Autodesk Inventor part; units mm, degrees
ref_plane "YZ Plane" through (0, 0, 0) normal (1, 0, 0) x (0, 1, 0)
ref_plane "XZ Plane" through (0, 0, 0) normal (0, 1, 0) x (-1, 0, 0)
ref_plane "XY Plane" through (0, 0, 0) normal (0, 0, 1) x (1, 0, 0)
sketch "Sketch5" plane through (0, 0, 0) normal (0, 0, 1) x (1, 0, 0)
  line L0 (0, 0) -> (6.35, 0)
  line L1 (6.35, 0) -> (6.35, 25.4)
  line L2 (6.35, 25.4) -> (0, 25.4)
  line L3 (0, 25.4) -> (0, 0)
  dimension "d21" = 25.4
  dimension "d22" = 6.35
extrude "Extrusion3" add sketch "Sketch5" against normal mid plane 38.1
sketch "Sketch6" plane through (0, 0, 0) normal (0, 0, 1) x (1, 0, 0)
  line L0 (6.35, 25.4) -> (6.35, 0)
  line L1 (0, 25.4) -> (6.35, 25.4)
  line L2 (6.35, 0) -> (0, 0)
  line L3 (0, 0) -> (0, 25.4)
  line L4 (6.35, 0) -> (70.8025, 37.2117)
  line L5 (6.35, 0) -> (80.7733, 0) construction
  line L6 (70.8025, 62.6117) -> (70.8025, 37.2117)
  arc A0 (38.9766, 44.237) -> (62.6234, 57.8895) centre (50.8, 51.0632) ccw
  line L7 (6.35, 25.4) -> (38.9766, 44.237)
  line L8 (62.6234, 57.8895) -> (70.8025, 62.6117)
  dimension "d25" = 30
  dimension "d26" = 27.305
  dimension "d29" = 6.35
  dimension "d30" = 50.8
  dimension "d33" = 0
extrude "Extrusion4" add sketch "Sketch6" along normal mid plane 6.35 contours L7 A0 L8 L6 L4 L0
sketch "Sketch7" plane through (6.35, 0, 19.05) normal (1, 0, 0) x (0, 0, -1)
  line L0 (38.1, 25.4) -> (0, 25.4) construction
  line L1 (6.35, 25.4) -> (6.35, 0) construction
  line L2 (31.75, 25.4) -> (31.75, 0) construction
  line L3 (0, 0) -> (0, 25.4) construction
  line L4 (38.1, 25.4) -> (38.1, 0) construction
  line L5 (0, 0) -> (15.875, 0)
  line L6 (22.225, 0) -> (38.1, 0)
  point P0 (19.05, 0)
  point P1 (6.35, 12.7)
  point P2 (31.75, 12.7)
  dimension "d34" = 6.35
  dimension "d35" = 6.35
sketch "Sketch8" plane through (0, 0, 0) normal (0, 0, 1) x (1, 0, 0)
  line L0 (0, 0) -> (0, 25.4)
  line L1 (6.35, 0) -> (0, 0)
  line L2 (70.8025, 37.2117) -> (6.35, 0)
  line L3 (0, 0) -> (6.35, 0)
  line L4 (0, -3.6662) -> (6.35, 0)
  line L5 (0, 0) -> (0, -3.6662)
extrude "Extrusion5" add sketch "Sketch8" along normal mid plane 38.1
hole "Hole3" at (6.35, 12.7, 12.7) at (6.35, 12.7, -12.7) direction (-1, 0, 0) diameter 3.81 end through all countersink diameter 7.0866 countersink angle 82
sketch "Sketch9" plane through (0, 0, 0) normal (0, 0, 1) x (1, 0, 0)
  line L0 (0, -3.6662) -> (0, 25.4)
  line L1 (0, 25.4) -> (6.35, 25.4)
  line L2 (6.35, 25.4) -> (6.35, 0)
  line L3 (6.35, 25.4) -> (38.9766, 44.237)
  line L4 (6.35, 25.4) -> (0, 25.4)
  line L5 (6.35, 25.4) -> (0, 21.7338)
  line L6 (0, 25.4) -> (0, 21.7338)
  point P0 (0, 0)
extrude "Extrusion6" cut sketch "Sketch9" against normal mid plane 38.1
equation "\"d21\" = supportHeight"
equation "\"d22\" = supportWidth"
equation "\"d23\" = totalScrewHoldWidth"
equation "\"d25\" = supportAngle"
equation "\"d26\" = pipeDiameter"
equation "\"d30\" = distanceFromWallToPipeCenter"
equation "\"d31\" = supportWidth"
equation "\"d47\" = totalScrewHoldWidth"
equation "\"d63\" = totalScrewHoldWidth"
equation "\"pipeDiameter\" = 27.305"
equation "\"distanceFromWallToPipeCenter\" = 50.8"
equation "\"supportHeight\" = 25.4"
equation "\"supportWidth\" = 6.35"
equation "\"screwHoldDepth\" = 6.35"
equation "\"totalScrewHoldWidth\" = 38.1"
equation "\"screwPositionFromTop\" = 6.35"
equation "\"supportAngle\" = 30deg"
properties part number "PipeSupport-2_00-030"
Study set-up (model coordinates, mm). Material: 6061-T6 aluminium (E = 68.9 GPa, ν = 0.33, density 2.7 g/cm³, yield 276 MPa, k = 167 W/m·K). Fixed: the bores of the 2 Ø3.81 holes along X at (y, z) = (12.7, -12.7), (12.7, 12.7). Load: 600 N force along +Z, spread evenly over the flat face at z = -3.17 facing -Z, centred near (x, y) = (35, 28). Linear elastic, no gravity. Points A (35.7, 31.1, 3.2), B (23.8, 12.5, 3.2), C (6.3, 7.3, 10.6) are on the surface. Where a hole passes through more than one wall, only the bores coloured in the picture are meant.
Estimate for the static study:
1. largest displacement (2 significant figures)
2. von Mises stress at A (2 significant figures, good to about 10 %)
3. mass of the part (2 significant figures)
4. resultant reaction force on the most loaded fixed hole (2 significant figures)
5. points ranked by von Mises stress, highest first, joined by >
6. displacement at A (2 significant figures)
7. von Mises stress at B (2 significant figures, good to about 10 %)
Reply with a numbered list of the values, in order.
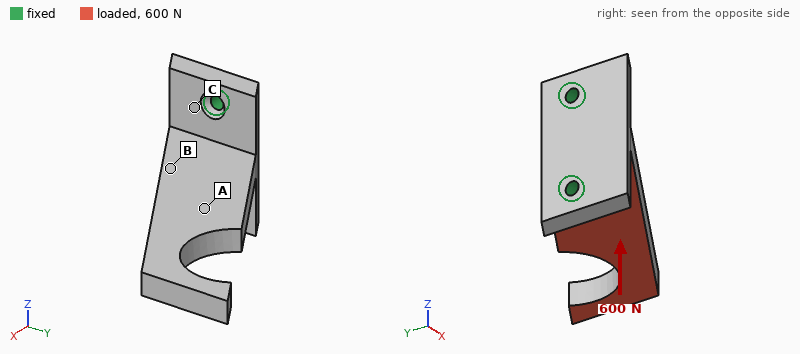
1. 1.0 mm
2. 35 MPa
3. 39 g
4. 1.0 kN
5. B > A > C
6. 0.29 mm
7. 76 MPa
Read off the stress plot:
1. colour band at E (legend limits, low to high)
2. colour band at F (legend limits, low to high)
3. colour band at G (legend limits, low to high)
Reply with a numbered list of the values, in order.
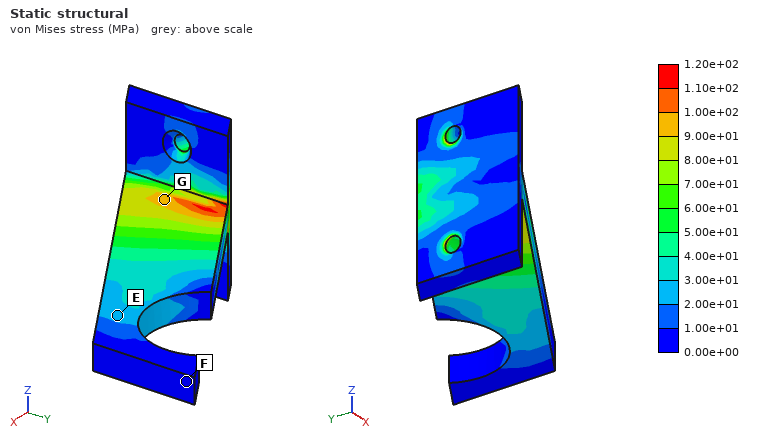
1. 2.00e+01 to 3.00e+01 MPa
2. 0.00e+00 to 1.00e+01 MPa
3. 9.00e+01 to 1.00e+02 MPa
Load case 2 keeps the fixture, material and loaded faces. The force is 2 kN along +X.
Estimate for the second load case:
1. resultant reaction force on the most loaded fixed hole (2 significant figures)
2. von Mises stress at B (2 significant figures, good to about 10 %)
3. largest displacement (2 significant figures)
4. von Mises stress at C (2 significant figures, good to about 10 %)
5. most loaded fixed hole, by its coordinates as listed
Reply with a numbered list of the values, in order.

1. 1.4 kN
2. 47 MPa
3. 0.73 mm
4. 44 MPa
5. (12.7, -12.7)
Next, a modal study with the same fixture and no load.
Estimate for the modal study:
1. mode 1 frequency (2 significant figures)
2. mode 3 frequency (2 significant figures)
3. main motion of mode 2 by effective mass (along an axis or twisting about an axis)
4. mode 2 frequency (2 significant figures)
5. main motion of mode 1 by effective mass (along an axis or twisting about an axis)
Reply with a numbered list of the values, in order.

1. 1100 Hz
2. 4200 Hz
3. along Y
4. 1700 Hz
5. along Z
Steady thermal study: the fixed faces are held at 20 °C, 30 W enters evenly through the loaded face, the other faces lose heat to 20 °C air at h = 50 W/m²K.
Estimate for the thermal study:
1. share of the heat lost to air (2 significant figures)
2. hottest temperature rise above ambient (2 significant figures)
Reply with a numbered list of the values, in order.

1. 16 %
2. 49 K
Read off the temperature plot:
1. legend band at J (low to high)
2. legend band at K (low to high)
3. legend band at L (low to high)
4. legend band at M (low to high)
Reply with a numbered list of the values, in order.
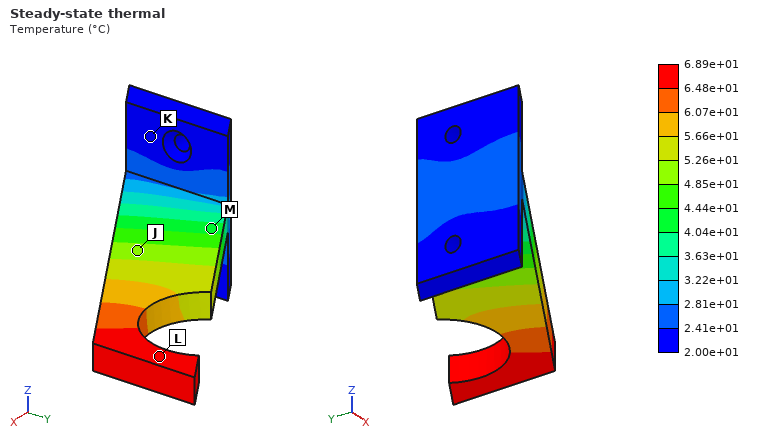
1. 4.85e+01 to 5.26e+01 °C
2. 2.00e+01 to 2.41e+01 °C
3. 6.48e+01 to 6.89e+01 °C
4. 4.04e+01 to 4.44e+01 °C
